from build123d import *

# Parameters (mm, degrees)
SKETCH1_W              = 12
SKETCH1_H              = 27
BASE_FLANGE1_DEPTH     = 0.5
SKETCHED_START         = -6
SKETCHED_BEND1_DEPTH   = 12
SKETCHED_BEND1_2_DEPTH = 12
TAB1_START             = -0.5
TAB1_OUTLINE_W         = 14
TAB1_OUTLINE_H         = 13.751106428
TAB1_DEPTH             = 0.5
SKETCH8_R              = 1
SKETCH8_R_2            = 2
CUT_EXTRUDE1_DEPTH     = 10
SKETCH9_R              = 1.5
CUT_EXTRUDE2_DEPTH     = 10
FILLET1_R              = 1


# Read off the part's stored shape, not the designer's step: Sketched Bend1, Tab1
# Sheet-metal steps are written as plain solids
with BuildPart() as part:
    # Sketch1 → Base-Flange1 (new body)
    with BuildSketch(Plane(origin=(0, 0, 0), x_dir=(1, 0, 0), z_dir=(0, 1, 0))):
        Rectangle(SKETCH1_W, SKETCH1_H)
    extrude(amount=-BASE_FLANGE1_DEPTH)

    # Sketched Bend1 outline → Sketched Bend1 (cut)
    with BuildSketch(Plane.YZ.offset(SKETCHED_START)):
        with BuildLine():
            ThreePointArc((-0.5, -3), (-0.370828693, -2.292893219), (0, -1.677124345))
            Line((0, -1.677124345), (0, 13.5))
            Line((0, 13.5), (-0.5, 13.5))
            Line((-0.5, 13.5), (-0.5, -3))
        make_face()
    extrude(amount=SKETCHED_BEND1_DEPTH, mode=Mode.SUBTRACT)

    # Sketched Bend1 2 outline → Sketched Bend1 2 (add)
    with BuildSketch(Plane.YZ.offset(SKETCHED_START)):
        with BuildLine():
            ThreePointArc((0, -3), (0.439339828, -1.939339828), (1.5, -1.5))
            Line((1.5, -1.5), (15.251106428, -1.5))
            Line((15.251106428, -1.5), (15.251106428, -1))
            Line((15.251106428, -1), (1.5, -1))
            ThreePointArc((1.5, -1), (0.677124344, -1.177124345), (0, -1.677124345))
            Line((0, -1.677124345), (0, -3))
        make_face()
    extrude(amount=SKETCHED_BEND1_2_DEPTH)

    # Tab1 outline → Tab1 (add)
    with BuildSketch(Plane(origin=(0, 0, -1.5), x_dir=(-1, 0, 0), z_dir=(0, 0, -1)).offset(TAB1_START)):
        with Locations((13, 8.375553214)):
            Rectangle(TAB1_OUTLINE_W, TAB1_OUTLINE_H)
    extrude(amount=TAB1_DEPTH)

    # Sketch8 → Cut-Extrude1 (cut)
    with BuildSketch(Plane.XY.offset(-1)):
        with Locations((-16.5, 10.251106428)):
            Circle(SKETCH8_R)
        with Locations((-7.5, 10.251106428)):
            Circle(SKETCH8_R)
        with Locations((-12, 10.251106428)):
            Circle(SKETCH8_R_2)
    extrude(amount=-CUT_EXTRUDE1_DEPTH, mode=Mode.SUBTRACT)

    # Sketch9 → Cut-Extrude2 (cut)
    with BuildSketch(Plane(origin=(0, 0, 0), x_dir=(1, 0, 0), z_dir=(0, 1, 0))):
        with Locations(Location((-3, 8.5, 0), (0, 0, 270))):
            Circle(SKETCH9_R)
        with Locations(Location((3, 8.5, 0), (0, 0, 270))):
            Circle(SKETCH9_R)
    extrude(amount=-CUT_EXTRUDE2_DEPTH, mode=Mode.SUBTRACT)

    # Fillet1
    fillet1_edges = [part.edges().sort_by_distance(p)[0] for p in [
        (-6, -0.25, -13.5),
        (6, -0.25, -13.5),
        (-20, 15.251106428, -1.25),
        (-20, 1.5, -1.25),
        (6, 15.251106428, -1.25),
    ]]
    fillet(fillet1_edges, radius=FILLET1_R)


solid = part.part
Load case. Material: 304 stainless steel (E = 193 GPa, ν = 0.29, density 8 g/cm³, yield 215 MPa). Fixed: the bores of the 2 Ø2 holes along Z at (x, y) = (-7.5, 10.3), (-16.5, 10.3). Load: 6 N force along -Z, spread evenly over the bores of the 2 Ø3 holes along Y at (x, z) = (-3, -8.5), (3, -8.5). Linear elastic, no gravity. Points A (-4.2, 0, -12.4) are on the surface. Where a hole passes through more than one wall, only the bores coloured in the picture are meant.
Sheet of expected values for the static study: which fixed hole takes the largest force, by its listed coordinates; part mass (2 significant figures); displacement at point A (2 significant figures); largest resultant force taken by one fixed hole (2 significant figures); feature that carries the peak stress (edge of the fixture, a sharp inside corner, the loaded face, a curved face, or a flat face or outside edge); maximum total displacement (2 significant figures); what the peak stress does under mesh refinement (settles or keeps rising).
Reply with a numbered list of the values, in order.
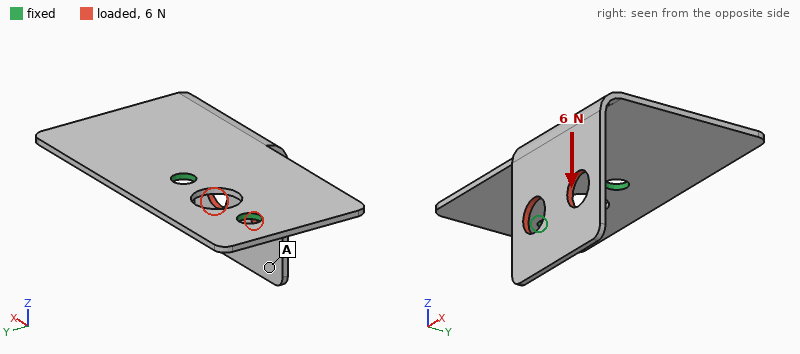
1. (-7.5, 10.3)
2. 1.9 g
3. 0.20 mm
4. 7.4 N
5. edge of the fixture
6. 0.28 mm
7. keeps rising
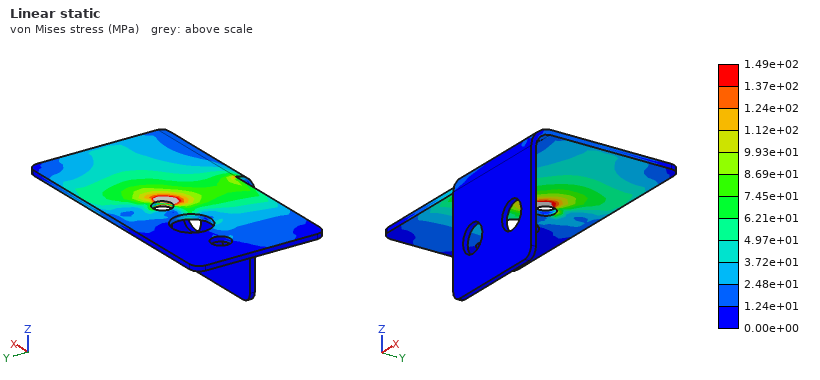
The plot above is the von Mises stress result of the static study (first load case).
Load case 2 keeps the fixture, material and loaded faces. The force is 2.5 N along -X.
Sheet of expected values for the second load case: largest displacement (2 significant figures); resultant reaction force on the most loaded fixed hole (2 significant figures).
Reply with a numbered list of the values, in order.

1. 87 µm
2. 2.6 N
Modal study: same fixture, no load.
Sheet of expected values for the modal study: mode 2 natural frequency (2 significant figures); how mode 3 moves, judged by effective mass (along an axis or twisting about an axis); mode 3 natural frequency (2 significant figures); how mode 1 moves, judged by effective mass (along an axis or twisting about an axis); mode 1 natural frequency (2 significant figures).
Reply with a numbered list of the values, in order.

1. 1600 Hz
2. along Z
3. 3100 Hz
4. along Z
5. 970 Hz
